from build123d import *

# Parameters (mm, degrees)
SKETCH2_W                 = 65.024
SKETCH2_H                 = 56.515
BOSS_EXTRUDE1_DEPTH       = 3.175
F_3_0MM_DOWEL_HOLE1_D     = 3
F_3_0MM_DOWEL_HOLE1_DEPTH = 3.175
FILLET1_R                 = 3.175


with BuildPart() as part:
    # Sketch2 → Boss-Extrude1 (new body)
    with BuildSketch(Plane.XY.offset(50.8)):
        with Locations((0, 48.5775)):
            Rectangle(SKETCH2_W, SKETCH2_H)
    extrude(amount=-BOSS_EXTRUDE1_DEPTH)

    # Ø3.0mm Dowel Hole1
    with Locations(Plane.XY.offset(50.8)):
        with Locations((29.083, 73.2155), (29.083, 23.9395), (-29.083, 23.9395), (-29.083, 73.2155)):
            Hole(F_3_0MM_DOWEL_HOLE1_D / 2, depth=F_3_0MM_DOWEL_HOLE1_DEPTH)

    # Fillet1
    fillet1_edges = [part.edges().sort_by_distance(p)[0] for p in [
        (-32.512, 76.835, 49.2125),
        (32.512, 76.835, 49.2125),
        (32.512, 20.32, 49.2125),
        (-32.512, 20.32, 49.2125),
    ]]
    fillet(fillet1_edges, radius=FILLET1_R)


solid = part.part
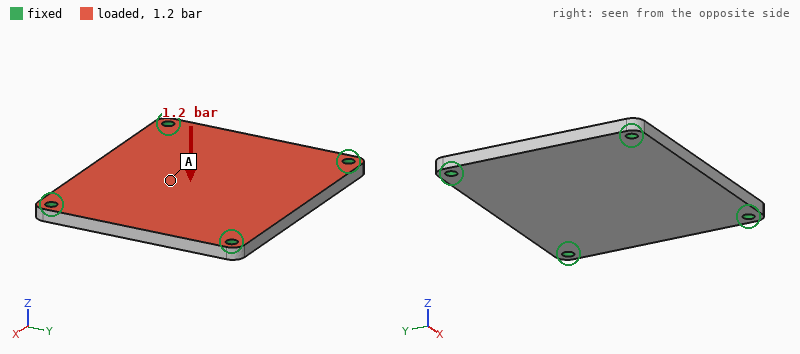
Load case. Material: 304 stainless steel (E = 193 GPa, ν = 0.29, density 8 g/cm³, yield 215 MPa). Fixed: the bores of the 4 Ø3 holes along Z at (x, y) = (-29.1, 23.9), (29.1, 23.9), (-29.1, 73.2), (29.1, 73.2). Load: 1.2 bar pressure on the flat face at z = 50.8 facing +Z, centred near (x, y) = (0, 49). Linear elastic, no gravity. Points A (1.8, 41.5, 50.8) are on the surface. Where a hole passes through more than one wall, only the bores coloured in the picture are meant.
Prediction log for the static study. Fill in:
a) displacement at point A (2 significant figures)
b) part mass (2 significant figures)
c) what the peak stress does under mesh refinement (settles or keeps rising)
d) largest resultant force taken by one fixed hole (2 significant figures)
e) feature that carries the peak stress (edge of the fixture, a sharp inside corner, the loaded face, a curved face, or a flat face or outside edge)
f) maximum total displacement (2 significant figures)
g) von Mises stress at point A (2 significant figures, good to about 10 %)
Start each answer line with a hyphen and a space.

- 15 µm
- 92 g
- keeps rising
- 110 N
- edge of the fixture
- 15 µm
- 12 MPa
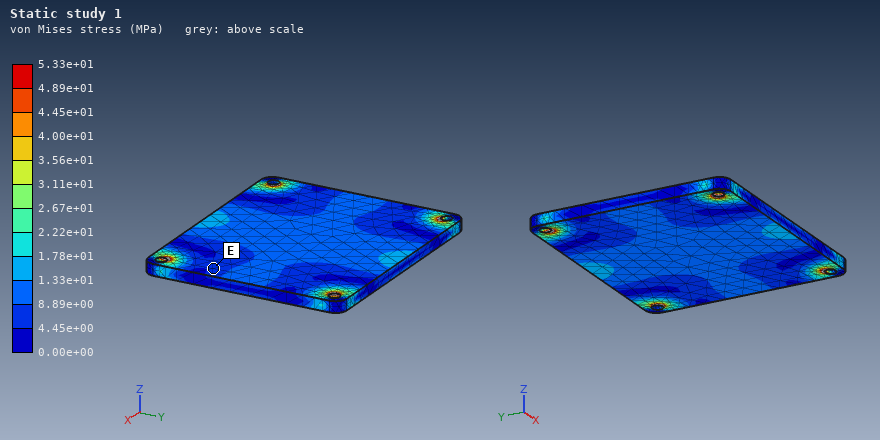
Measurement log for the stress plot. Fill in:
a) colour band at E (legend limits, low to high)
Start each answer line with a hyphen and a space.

- 4.45e+00 to 8.89e+00 MPa
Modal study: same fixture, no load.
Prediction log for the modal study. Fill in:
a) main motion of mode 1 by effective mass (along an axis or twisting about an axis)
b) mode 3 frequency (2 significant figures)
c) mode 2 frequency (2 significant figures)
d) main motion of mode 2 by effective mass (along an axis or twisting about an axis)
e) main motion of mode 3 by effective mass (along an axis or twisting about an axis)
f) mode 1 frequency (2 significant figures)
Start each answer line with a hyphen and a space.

- along Z
- 6600 Hz
- 5500 Hz
- twisting about X
- twisting about Y
- 3300 Hz
